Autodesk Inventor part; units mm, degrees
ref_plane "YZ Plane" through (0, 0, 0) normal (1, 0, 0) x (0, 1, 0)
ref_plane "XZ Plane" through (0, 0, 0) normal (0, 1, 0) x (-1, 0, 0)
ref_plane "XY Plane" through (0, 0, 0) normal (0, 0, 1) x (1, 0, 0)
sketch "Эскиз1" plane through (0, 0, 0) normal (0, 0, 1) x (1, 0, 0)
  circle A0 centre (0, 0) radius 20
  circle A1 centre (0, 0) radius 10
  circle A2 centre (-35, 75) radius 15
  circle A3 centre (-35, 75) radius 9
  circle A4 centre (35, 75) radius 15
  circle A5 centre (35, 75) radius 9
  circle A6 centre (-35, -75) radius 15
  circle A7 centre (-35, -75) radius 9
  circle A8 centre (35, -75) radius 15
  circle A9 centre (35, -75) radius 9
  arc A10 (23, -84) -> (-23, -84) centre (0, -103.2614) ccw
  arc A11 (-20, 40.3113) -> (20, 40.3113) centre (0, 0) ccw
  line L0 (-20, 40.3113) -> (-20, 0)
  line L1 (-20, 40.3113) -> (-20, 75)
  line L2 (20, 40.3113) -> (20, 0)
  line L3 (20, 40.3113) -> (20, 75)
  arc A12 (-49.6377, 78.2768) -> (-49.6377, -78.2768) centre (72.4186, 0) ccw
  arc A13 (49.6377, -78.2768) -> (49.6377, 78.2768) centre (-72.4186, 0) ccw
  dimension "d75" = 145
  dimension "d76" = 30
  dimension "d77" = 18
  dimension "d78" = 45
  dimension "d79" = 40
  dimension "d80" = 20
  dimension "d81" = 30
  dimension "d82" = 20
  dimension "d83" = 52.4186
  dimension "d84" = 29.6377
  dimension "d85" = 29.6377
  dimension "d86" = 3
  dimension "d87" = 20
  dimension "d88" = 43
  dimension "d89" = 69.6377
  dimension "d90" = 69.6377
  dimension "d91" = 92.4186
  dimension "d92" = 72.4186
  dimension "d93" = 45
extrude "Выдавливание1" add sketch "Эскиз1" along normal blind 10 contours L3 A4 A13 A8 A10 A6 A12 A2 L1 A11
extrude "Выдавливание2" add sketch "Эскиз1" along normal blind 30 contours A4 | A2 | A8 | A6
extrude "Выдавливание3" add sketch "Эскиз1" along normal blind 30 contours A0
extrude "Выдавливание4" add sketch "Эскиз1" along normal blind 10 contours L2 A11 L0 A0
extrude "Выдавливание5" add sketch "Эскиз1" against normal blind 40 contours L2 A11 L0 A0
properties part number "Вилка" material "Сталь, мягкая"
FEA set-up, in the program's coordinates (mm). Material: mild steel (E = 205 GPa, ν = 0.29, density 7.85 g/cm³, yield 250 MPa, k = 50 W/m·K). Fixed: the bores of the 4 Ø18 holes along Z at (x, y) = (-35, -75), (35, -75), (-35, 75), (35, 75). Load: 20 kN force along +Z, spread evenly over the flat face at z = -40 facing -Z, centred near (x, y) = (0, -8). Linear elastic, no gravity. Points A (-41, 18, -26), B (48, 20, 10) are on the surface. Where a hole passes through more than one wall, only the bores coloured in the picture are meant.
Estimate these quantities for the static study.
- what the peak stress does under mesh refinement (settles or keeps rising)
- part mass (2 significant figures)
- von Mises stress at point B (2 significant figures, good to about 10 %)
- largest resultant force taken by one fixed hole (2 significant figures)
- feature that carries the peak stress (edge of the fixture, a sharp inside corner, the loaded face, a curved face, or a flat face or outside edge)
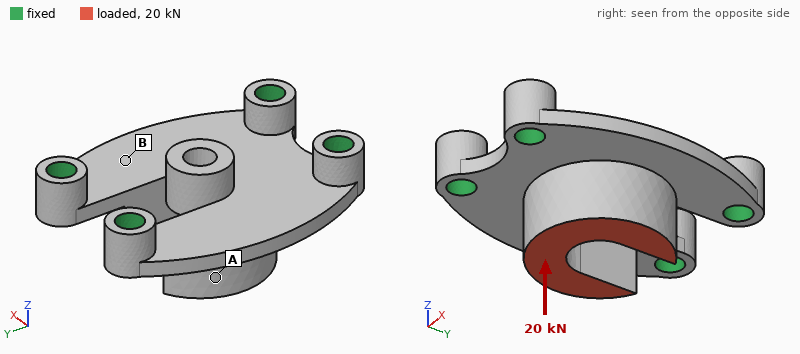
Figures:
keeps rising
3.1 kg
34 MPa
6.6 kN
a sharp inside corner
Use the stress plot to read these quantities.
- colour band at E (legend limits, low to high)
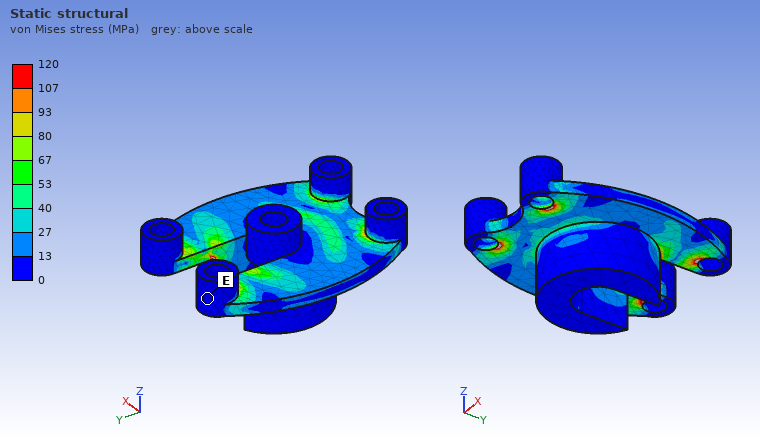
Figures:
0 to 13 MPa
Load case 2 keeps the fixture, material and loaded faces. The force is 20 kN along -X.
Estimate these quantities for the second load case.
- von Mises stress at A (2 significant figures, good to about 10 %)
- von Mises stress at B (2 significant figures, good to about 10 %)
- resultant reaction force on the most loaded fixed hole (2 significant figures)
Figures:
22 MPa
48 MPa
13 kN
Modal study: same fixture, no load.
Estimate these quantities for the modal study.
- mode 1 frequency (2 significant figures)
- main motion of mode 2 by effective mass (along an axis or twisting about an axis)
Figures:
2200 Hz
along Z
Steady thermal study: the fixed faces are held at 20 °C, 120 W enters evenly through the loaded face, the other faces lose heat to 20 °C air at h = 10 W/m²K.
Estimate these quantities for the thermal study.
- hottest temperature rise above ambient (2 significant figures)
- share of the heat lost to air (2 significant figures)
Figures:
70 K
17 %
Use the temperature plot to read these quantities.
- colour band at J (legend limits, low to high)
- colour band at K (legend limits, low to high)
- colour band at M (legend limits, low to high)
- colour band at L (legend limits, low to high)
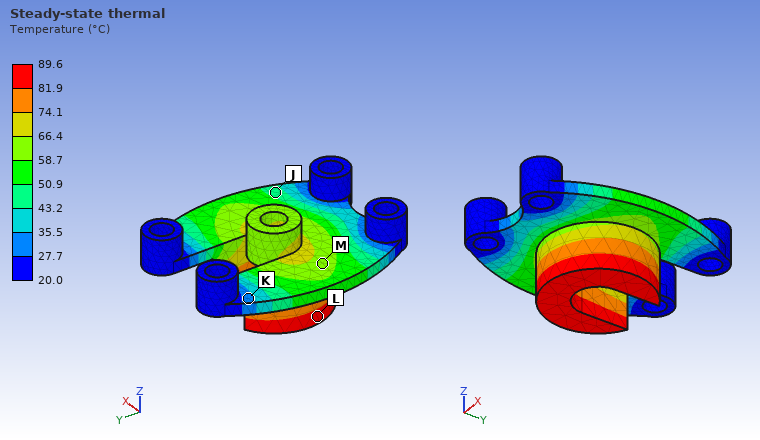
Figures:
43.2 to 50.9 °C
27.7 to 35.5 °C
58.7 to 66.4 °C
81.9 to 89.6 °C
